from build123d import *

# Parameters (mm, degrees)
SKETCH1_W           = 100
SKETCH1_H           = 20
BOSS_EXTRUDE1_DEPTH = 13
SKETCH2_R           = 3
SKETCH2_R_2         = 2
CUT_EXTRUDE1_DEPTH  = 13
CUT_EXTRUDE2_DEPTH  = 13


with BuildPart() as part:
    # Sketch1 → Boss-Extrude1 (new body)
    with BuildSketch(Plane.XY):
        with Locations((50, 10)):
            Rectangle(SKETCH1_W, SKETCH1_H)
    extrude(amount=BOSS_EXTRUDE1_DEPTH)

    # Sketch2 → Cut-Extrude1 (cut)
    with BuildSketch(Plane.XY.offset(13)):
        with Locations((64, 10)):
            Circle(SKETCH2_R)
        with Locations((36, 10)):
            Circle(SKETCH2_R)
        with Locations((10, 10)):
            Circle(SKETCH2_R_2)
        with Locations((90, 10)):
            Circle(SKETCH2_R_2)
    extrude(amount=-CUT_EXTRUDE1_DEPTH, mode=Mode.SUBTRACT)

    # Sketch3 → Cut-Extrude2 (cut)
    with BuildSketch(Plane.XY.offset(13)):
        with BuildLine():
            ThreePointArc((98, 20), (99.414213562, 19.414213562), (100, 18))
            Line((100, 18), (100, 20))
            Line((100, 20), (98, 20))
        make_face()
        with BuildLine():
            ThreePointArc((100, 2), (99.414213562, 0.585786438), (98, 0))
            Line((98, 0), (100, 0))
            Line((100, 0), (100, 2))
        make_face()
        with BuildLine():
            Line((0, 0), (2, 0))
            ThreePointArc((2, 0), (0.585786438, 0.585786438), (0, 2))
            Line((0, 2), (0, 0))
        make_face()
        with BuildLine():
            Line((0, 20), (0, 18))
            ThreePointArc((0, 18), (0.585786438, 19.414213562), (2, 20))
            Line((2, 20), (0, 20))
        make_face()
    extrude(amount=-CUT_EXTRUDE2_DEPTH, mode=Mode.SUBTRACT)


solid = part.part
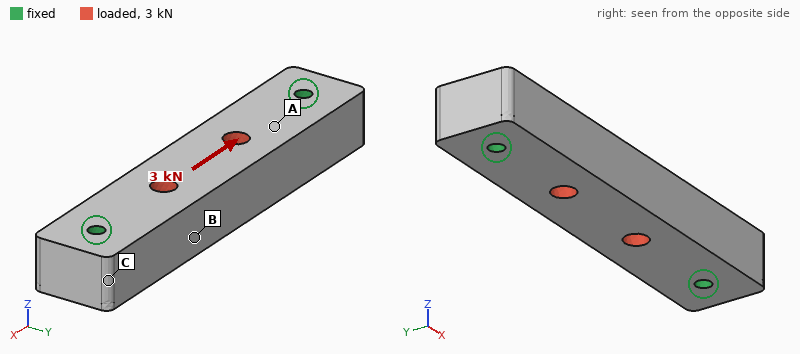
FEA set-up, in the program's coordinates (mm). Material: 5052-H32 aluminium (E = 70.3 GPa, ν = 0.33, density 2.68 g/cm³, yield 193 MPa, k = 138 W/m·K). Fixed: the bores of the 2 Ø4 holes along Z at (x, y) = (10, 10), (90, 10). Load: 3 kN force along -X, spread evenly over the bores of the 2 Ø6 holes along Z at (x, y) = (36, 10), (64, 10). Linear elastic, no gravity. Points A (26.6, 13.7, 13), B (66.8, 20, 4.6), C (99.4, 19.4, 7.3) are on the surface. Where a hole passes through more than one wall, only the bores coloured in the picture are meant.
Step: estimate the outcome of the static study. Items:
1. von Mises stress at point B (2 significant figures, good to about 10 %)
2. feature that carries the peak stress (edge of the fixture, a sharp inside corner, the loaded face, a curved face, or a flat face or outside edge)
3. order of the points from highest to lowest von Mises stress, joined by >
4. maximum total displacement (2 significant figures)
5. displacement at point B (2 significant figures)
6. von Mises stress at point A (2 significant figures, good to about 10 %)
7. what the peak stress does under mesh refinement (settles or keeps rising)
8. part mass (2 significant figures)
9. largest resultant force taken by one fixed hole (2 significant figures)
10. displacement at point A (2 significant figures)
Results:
3.3 MPa
edge of the fixture
A > B > C
3.2 µm
2.1 µm
6.5 MPa
keeps rising
67 g
1.5 kN
1.8 µm
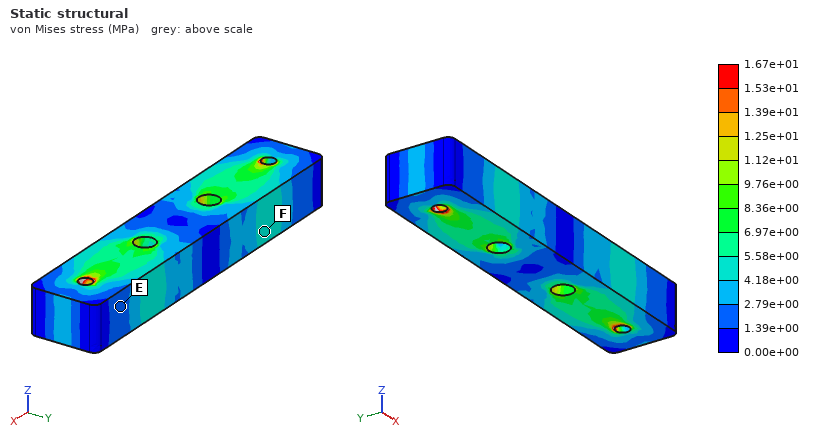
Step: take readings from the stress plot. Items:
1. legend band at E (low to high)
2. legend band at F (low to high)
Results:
1.39e+00 to 2.79e+00 MPa
4.18e+00 to 5.58e+00 MPa
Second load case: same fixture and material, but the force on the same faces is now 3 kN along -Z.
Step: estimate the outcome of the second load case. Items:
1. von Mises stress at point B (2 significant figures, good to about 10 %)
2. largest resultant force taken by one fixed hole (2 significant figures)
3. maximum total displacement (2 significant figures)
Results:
15 MPa
1.5 kN
35 µm
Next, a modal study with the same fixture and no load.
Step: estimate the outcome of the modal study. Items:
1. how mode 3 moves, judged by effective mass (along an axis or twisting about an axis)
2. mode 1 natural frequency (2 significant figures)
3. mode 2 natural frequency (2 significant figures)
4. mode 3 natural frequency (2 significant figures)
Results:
twisting about X
8600 Hz
8600 Hz
16 kHz
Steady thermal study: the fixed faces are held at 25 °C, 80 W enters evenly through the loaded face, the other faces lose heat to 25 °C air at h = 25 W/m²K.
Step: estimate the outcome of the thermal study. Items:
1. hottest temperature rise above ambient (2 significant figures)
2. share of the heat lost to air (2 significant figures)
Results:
34 K
3.4 %
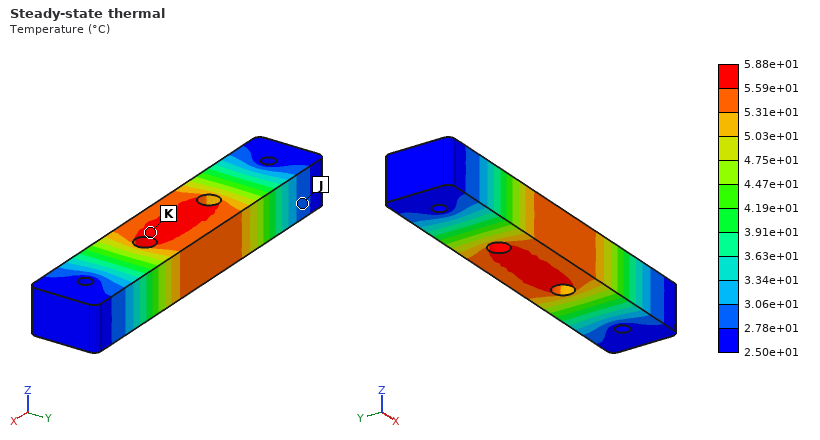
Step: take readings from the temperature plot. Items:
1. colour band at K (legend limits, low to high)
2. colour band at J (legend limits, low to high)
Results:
5.59e+01 to 5.88e+01 °C
2.78e+01 to 3.06e+01 °C
